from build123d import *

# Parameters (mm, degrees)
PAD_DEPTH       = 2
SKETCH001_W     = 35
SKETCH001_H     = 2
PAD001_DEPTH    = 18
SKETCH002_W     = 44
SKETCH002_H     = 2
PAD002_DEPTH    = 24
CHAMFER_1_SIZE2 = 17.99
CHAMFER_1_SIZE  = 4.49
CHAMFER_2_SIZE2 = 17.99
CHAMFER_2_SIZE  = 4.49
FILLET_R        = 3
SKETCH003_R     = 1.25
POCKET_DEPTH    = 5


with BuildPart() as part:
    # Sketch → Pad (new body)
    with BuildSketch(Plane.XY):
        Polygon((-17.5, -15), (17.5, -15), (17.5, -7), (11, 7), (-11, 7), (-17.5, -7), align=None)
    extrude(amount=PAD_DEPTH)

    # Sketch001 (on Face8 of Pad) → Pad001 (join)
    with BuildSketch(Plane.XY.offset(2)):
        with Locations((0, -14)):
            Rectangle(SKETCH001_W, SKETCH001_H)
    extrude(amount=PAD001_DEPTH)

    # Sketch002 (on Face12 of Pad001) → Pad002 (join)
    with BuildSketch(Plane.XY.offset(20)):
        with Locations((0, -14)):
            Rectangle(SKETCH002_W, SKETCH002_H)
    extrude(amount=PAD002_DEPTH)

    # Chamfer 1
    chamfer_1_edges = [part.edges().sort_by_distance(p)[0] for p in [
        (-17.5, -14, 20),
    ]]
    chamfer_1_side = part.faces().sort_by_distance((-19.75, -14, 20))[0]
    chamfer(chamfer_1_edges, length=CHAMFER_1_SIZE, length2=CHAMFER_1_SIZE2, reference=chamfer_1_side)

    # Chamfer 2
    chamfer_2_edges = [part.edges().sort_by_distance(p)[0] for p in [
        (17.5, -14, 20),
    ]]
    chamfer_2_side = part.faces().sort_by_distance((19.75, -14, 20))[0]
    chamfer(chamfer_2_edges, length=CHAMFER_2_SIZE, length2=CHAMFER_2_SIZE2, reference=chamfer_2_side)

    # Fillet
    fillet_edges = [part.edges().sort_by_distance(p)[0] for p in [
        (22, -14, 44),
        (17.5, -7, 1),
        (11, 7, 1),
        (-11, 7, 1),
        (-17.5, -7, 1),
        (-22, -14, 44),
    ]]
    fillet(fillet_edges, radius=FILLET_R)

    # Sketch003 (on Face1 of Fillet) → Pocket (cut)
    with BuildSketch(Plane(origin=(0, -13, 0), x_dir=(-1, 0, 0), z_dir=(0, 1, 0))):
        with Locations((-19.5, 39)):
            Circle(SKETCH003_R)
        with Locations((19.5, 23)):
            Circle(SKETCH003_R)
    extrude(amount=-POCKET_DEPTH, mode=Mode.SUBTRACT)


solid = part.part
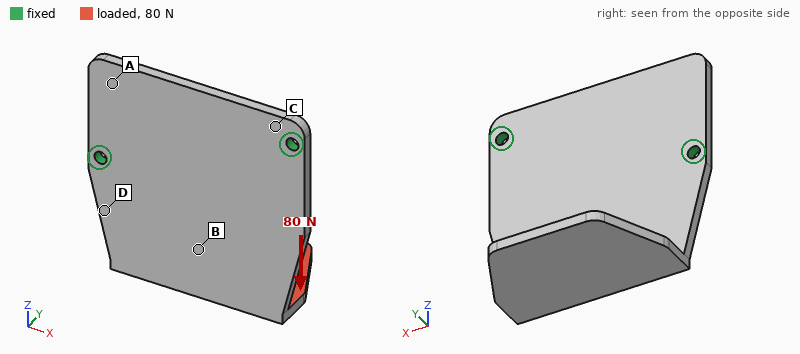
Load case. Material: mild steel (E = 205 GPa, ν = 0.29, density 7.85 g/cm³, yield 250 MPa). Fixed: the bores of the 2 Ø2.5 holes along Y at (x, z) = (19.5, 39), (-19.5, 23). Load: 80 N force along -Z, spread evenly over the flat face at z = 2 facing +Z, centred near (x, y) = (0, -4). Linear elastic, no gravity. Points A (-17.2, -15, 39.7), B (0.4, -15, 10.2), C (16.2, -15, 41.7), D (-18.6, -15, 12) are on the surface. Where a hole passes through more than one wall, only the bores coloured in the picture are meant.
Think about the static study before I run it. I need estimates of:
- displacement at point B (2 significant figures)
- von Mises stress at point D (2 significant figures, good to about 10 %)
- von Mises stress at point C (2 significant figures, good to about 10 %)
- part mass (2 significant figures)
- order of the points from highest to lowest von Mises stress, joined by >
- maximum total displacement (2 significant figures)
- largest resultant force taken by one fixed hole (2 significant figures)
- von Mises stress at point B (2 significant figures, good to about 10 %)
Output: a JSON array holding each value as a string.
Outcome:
["0.034 mm", "39 MPa", "14 MPa", "38 g", "D > B > C > A", "0.13 mm", "43 N", "27 MPa"]
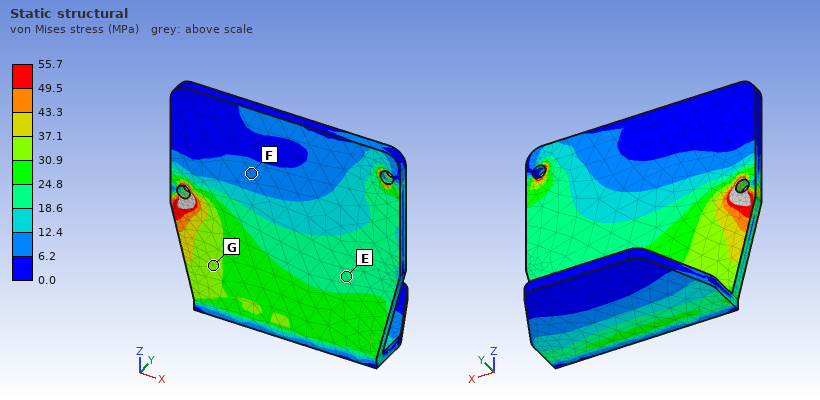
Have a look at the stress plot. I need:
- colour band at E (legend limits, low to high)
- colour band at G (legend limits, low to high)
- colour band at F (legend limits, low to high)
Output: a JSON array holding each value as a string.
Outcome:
["18.6 to 24.8 MPa", "30.9 to 37.1 MPa", "6.2 to 12.4 MPa"]
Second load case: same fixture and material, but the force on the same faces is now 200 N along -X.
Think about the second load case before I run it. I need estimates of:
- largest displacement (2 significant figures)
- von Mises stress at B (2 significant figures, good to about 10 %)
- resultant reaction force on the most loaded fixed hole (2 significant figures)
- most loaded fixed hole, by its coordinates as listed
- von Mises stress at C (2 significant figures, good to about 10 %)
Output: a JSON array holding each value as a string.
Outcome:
["0.16 mm", "40 MPa", "200 N", "(-19.5, 23)", "30 MPa"]
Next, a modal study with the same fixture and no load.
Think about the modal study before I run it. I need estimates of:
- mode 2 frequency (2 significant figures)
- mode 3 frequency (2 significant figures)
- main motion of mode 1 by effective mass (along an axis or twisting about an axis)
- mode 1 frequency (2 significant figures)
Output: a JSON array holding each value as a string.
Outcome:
["2100 Hz", "3100 Hz", "along Y", "860 Hz"]
